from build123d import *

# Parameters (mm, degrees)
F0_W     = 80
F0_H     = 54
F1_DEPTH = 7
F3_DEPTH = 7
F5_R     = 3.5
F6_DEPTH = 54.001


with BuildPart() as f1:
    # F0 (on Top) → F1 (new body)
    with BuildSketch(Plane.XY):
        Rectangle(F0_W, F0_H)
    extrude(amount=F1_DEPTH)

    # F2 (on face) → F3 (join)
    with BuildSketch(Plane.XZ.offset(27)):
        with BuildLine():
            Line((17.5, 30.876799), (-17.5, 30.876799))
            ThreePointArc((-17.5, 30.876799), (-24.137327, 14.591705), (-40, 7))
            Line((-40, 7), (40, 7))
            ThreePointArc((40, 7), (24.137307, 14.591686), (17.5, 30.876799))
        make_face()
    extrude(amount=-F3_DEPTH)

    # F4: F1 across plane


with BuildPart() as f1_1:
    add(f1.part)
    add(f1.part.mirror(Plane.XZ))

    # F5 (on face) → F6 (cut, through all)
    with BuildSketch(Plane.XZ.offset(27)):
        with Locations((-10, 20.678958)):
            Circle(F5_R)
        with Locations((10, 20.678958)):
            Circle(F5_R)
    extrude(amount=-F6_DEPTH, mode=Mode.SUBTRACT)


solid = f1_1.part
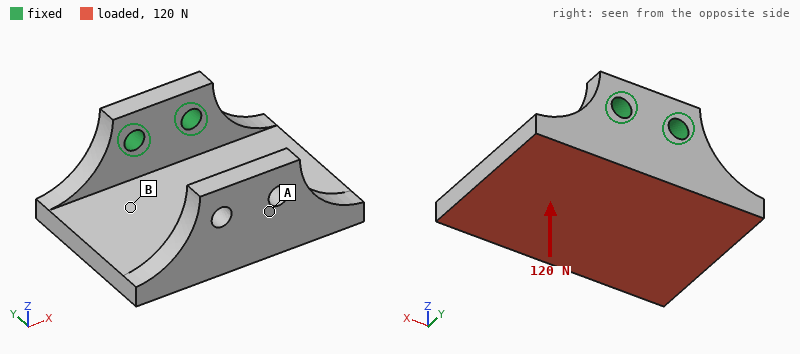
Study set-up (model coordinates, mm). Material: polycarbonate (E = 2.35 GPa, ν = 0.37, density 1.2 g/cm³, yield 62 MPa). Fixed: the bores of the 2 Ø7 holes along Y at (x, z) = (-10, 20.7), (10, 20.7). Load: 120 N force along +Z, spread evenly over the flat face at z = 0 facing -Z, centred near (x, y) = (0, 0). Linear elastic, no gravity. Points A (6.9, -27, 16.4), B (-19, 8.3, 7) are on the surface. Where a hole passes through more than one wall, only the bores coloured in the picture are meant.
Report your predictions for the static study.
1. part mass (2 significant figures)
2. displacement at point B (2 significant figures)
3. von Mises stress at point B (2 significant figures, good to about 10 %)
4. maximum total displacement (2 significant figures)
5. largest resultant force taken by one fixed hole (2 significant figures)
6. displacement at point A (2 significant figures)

53 g
0.23 mm
2.0 MPa
1.0 mm
60 N
0.92 mm
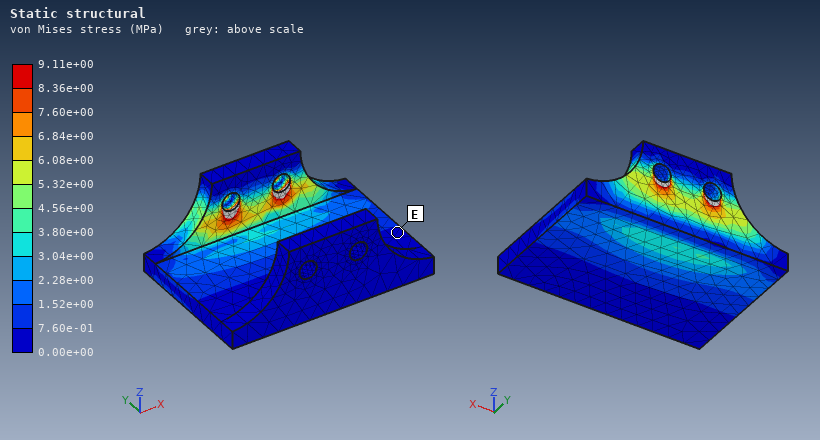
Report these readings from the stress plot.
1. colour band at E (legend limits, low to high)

0.00e+00 to 7.60e-01 MPa
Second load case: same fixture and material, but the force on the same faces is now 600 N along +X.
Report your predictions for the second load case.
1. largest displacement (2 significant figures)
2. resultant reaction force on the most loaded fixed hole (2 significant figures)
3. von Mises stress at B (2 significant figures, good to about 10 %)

1.1 mm
720 N
4.6 MPa
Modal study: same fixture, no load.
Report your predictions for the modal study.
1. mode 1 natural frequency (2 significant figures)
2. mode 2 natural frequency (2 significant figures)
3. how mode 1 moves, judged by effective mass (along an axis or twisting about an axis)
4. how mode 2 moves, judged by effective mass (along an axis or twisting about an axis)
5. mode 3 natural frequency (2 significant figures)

280 Hz
470 Hz
along Z
along X
820 Hz
